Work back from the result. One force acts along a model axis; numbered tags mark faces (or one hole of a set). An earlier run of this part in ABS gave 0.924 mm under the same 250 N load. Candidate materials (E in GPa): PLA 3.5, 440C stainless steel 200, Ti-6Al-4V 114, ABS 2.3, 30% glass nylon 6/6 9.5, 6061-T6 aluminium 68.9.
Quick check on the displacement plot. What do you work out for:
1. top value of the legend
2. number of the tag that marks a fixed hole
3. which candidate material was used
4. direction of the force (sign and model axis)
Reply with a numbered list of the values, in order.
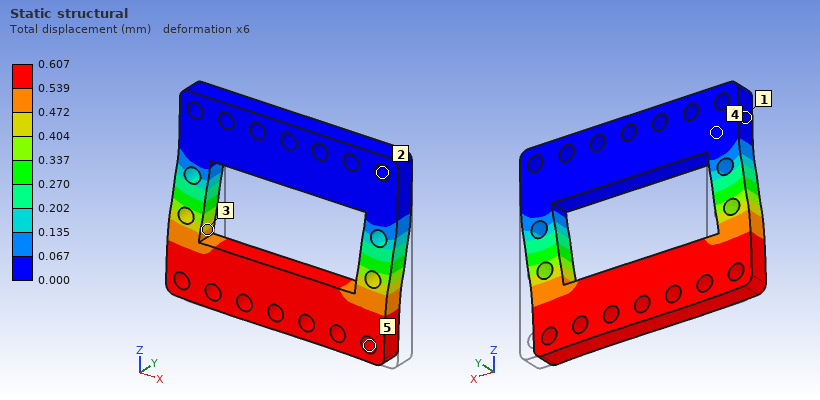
1. 0.607 mm
2. 2
3. PLA
4. -X
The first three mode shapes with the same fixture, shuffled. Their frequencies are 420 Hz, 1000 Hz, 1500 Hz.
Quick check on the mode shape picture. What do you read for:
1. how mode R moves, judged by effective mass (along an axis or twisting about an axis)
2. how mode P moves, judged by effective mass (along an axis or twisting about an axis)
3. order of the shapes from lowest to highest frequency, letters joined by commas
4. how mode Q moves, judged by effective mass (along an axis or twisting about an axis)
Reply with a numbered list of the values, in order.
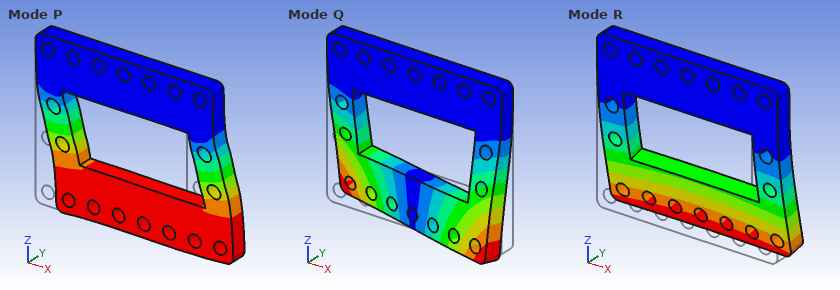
1. along Y
2. along X
3. R, Q, P
4. twisting about Z
